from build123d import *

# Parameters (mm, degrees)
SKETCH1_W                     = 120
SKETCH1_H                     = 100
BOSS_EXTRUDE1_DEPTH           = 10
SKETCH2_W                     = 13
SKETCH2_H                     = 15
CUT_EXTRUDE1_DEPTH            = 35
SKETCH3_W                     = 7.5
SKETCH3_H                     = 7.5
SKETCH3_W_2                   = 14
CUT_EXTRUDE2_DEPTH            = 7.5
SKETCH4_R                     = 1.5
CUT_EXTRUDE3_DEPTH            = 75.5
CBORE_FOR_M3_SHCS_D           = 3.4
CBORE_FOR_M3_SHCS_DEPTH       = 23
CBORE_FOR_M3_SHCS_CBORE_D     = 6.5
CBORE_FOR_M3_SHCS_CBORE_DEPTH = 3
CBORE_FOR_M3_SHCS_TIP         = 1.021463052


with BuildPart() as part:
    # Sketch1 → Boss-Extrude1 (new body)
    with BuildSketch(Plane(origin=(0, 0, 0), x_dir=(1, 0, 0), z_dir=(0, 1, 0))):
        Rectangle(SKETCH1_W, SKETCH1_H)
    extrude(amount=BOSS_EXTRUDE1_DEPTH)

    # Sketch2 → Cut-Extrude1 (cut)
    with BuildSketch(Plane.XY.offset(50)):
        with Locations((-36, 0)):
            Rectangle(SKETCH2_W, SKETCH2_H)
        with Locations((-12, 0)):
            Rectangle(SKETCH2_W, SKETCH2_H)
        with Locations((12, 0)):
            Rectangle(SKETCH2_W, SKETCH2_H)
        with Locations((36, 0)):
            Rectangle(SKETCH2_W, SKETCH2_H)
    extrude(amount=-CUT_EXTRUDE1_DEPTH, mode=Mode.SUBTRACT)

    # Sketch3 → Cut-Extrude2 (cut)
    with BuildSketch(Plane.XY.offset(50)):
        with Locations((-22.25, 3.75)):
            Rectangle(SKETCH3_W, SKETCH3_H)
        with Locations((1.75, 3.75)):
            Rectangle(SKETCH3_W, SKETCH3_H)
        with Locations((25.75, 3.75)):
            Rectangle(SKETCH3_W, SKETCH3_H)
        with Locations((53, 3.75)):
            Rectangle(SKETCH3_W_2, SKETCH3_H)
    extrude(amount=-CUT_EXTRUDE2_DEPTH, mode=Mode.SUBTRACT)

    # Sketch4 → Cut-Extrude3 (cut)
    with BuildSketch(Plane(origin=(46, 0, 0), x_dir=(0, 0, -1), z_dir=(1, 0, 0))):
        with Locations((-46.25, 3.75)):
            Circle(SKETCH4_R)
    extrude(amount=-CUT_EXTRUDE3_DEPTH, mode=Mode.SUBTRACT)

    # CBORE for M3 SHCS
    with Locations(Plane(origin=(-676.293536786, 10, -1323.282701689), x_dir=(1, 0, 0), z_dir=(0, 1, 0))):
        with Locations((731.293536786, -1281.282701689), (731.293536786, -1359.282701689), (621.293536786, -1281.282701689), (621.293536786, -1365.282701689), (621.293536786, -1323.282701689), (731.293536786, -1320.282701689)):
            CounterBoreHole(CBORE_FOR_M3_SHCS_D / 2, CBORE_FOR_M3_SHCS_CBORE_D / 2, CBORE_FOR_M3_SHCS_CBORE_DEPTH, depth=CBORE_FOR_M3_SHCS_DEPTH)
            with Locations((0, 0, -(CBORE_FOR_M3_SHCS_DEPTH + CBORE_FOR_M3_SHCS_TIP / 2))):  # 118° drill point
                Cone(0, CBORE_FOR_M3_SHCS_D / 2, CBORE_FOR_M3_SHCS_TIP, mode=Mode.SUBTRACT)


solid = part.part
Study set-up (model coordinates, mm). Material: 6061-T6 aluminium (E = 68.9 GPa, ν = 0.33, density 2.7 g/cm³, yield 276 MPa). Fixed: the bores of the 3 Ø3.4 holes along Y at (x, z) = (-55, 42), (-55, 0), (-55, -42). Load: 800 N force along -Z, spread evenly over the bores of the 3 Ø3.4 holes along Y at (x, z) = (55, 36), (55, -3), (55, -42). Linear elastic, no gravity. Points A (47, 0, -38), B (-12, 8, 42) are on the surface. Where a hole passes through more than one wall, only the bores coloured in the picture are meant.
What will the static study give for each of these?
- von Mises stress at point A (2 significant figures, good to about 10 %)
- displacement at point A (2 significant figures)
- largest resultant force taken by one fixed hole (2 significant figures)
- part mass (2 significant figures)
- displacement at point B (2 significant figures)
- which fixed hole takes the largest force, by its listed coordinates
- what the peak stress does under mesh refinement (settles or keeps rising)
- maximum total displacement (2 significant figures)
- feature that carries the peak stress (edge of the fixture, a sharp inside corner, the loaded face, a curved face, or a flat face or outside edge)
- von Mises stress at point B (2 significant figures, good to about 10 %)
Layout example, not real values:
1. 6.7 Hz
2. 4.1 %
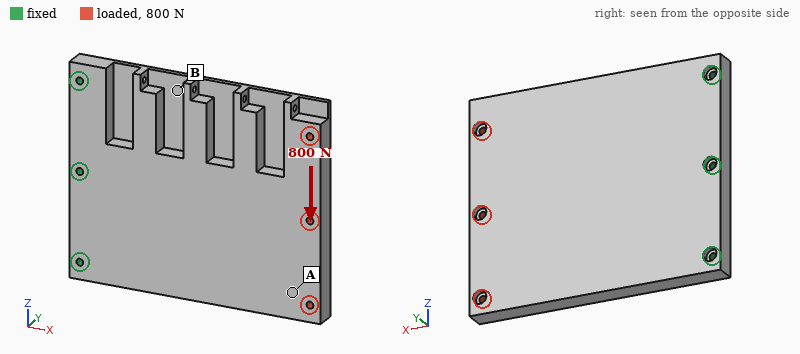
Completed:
1. 2.3 MPa
2. 44 µm
3. 1.4 kN
4. 280 g
5. 9.8 µm
6. (-55, -42)
7. keeps rising
8. 54 µm
9. edge of the fixture
10. 8.4 MPa
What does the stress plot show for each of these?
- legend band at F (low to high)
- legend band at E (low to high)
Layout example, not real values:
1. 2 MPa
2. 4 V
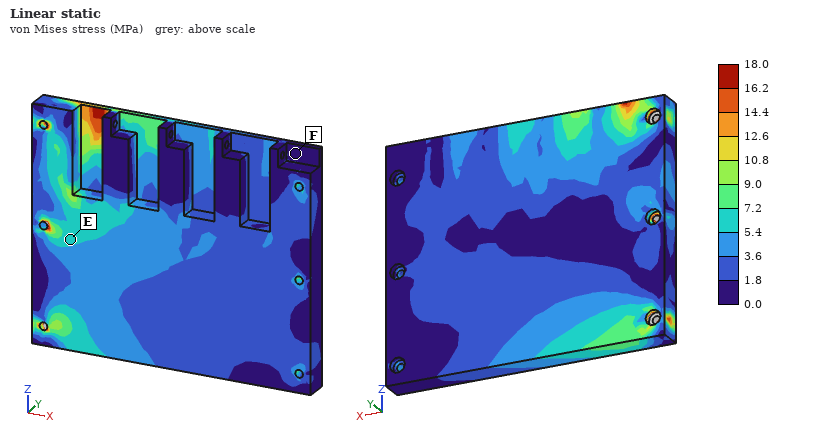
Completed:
1. 0.0 to 1.8 MPa
2. 5.4 to 7.2 MPa
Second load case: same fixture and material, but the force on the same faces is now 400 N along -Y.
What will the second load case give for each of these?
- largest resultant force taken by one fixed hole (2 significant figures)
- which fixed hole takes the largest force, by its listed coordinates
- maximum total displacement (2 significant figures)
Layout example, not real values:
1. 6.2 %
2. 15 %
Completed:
1. 1.2 kN
2. (-55, 0)
3. 0.71 mm
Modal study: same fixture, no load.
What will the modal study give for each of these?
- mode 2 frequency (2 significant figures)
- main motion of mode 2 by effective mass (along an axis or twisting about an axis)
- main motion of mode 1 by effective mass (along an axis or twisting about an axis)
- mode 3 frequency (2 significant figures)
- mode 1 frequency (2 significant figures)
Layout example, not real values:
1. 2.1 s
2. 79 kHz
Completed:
1. 1400 Hz
2. twisting about X
3. along Y
4. 2700 Hz
5. 450 Hz
